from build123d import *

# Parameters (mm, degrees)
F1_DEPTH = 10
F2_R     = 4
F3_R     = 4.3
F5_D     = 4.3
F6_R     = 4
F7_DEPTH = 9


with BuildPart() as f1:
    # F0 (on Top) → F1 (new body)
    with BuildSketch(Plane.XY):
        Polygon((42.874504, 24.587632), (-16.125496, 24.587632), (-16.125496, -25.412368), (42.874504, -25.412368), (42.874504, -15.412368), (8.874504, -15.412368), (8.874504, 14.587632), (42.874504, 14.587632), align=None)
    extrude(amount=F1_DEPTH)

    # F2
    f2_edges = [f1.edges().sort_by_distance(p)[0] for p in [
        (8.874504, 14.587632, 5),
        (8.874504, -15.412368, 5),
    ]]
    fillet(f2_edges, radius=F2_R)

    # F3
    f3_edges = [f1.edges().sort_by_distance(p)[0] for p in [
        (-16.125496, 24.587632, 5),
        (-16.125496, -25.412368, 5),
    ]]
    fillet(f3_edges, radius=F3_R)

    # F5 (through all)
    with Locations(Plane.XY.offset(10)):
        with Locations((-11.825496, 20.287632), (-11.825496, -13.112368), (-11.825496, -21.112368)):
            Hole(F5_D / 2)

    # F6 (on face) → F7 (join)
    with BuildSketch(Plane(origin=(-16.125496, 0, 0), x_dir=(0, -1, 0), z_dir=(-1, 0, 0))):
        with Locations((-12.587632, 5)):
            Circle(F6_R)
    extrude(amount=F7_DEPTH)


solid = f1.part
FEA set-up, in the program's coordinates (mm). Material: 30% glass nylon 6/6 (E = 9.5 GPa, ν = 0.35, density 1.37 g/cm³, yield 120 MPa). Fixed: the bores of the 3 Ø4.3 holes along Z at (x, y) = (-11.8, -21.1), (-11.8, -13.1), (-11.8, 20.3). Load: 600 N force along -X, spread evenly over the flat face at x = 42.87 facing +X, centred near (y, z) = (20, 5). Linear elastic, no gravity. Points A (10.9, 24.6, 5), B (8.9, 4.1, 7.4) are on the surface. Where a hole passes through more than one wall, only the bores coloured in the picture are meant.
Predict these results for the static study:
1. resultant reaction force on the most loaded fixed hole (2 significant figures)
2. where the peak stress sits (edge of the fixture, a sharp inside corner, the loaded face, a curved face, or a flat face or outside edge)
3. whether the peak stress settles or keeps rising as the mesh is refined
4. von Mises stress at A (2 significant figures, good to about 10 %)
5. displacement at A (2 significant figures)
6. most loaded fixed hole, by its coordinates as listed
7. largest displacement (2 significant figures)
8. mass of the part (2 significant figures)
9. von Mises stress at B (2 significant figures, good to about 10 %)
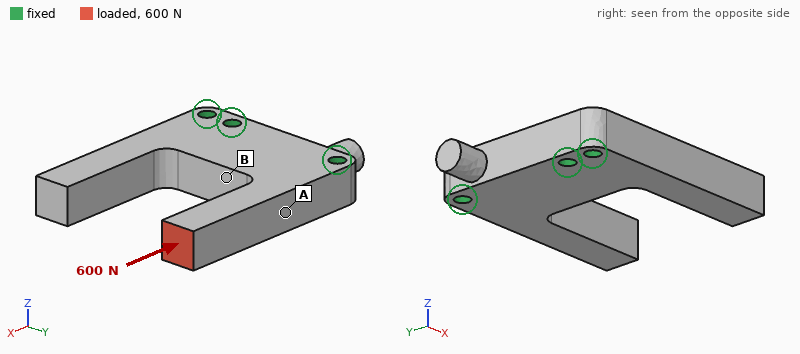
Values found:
580 N
edge of the fixture
keeps rising
6.6 MPa
18 µm
(-11.8, 20.3)
49 µm
26 g
1.1 MPa
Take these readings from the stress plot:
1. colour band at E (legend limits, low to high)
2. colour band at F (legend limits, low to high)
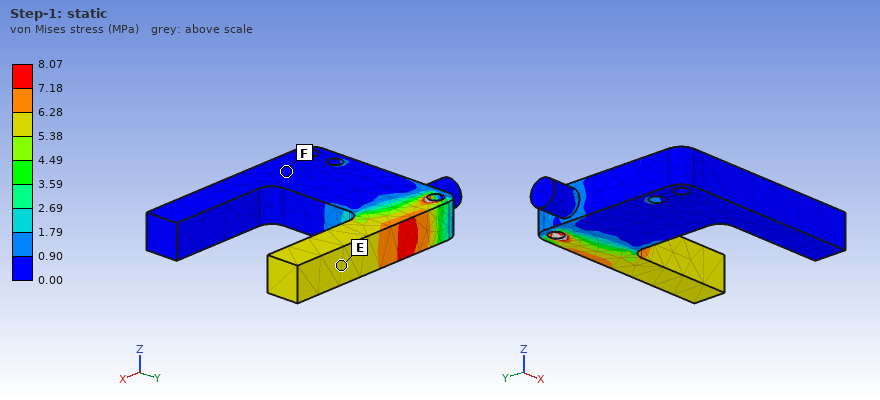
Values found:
5.38 to 6.28 MPa
0.00 to 0.90 MPa
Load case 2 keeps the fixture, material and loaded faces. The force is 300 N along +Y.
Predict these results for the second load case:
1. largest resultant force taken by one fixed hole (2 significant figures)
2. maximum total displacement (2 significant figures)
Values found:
460 N
0.76 mm
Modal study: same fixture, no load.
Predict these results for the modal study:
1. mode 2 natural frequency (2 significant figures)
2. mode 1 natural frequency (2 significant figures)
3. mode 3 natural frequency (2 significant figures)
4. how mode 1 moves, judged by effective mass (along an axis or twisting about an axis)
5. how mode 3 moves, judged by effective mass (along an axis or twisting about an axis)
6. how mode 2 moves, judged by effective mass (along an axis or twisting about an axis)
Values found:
1900 Hz
1700 Hz
2700 Hz
along Z
along Y
twisting about X
